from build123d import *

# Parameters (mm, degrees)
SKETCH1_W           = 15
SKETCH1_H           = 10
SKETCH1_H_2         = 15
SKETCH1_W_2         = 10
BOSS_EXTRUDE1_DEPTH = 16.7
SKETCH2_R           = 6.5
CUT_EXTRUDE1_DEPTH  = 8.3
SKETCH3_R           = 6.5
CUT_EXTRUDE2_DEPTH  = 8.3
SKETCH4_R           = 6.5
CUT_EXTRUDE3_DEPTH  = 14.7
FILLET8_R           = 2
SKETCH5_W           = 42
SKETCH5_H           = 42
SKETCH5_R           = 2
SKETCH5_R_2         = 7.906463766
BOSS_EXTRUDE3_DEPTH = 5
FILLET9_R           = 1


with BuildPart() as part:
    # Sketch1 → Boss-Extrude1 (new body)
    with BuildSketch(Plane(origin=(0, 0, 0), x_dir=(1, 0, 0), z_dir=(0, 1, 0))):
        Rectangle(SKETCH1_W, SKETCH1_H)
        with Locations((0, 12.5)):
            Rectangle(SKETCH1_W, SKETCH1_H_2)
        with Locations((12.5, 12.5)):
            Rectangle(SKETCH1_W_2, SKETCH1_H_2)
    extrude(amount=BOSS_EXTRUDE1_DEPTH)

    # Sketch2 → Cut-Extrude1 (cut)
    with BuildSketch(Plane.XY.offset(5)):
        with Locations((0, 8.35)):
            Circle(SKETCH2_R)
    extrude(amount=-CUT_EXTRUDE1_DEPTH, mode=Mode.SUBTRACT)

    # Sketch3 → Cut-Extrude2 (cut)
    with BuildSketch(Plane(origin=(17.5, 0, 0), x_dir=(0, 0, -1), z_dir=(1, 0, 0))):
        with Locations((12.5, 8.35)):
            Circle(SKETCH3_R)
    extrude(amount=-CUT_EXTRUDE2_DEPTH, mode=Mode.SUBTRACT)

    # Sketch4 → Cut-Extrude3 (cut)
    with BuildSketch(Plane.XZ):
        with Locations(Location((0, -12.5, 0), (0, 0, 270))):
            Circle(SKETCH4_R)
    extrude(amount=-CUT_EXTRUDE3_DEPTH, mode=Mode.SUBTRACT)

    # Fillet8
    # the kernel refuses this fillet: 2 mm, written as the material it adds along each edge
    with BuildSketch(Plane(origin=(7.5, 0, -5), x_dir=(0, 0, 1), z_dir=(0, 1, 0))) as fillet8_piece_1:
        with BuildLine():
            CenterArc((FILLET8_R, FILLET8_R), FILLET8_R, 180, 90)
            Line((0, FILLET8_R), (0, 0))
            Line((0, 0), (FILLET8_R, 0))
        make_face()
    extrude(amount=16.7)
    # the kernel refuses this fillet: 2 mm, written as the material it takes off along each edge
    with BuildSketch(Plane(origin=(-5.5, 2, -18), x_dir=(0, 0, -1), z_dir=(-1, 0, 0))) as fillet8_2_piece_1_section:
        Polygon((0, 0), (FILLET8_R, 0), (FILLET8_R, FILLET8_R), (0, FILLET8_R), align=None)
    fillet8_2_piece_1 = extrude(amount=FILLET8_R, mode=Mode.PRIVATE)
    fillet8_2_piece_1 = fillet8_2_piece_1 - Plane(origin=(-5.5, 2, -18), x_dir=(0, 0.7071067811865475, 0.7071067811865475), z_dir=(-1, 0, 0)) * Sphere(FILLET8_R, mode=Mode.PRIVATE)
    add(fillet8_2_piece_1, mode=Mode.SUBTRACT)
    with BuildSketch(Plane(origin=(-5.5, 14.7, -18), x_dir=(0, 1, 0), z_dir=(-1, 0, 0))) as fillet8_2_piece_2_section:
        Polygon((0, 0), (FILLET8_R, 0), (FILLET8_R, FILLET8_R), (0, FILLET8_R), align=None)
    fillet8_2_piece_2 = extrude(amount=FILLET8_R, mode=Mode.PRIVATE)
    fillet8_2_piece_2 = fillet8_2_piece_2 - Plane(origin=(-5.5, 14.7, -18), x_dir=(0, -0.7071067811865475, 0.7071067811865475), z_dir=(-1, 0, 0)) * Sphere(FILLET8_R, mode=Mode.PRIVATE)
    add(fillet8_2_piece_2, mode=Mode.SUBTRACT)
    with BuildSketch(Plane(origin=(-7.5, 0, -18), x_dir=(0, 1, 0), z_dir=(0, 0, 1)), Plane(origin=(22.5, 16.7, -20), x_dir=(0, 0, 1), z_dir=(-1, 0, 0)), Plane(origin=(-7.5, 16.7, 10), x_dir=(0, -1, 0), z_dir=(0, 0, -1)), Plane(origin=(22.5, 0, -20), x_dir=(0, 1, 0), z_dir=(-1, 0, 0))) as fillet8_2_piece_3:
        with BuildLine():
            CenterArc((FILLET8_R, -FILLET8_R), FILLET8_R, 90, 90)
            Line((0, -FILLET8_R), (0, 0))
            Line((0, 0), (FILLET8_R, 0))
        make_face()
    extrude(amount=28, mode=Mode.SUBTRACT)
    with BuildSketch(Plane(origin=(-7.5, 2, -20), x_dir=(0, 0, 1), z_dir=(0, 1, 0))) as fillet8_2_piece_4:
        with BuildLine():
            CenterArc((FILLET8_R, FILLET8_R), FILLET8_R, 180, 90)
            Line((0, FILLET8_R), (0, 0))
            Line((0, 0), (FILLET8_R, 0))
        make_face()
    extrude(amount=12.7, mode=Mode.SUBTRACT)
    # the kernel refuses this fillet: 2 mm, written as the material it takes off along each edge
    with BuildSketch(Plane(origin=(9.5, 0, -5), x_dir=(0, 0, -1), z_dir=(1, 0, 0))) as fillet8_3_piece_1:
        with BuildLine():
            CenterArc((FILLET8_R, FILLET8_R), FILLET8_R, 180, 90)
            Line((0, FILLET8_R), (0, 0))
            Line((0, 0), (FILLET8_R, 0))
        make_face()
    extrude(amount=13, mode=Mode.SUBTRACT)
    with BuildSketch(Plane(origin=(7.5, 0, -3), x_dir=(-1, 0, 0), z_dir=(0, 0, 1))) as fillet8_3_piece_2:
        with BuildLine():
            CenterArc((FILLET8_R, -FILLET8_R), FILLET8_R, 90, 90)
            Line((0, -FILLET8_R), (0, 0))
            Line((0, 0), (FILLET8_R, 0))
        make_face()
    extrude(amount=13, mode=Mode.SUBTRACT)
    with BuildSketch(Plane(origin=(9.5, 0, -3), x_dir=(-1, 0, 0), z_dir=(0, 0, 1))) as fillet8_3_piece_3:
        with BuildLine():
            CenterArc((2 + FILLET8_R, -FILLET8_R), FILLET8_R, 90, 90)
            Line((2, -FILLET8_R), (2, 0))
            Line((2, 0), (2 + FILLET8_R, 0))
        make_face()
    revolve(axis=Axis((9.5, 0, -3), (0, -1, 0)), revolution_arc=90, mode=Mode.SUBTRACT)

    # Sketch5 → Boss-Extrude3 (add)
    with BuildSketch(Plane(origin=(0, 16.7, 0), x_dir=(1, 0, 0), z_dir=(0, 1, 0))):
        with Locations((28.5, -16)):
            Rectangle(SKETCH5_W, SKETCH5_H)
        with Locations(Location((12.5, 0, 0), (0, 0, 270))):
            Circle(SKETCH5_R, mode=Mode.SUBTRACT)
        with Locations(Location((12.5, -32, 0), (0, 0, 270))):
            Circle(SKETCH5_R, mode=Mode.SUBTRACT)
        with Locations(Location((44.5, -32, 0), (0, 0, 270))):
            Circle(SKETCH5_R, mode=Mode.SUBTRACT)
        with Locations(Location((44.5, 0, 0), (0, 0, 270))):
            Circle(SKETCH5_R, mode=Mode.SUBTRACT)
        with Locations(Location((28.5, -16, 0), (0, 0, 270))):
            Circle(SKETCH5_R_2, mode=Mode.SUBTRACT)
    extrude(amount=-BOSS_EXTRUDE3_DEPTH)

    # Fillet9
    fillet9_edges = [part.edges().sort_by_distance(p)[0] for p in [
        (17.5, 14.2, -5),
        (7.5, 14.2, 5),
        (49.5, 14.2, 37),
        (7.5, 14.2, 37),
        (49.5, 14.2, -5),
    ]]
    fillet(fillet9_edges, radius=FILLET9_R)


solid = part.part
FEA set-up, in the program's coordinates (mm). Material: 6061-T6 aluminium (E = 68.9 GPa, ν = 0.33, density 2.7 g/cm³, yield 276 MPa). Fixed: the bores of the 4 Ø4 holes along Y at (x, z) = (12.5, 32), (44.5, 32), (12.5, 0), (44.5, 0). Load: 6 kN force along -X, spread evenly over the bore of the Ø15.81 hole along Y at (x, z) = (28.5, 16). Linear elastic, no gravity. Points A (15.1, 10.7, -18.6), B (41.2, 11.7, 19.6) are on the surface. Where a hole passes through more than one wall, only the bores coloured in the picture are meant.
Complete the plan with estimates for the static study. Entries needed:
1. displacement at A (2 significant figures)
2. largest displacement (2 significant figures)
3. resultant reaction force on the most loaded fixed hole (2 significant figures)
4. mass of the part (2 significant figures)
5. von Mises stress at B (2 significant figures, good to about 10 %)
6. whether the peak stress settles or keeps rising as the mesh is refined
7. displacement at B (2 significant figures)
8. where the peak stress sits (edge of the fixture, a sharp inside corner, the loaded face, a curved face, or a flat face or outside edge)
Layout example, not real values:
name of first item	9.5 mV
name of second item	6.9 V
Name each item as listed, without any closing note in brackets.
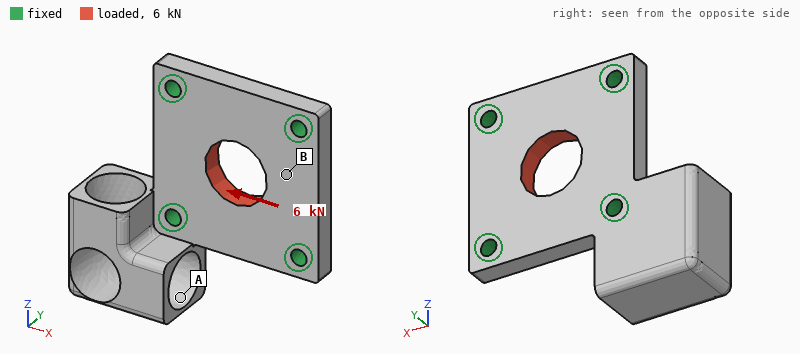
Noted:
displacement at A	2.4 µm
largest displacement	10.0 µm
resultant reaction force on the most loaded fixed hole	1.7 kN
mass of the part	33 g
von Mises stress at B	19 MPa
whether the peak stress settles or keeps rising as the mesh is refined	keeps rising
displacement at B	8.1 µm
where the peak stress sits	edge of the fixture
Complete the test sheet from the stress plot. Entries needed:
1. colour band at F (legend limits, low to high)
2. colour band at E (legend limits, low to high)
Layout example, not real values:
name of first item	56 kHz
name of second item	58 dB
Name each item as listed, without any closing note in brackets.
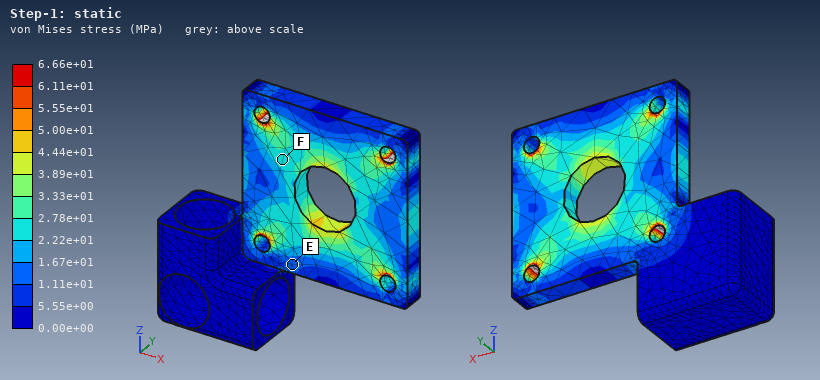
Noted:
colour band at F	2.22e+01 to 2.78e+01 MPa
colour band at E	1.11e+01 to 1.67e+01 MPa
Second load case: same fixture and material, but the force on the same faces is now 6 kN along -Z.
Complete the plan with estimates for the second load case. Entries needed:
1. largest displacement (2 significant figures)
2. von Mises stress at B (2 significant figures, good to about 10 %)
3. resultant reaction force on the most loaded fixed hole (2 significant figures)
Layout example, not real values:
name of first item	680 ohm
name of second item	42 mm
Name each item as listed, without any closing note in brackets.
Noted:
largest displacement	10 µm
von Mises stress at B	24 MPa
resultant reaction force on the most loaded fixed hole	1.7 kN
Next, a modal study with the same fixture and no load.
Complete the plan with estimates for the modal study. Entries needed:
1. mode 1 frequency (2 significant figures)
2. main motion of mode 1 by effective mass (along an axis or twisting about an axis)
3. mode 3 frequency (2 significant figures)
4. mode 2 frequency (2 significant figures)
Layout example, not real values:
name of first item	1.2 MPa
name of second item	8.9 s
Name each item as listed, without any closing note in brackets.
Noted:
mode 1 frequency	4500 Hz
main motion of mode 1 by effective mass	along Y
mode 3 frequency	9200 Hz
mode 2 frequency	6600 Hz
